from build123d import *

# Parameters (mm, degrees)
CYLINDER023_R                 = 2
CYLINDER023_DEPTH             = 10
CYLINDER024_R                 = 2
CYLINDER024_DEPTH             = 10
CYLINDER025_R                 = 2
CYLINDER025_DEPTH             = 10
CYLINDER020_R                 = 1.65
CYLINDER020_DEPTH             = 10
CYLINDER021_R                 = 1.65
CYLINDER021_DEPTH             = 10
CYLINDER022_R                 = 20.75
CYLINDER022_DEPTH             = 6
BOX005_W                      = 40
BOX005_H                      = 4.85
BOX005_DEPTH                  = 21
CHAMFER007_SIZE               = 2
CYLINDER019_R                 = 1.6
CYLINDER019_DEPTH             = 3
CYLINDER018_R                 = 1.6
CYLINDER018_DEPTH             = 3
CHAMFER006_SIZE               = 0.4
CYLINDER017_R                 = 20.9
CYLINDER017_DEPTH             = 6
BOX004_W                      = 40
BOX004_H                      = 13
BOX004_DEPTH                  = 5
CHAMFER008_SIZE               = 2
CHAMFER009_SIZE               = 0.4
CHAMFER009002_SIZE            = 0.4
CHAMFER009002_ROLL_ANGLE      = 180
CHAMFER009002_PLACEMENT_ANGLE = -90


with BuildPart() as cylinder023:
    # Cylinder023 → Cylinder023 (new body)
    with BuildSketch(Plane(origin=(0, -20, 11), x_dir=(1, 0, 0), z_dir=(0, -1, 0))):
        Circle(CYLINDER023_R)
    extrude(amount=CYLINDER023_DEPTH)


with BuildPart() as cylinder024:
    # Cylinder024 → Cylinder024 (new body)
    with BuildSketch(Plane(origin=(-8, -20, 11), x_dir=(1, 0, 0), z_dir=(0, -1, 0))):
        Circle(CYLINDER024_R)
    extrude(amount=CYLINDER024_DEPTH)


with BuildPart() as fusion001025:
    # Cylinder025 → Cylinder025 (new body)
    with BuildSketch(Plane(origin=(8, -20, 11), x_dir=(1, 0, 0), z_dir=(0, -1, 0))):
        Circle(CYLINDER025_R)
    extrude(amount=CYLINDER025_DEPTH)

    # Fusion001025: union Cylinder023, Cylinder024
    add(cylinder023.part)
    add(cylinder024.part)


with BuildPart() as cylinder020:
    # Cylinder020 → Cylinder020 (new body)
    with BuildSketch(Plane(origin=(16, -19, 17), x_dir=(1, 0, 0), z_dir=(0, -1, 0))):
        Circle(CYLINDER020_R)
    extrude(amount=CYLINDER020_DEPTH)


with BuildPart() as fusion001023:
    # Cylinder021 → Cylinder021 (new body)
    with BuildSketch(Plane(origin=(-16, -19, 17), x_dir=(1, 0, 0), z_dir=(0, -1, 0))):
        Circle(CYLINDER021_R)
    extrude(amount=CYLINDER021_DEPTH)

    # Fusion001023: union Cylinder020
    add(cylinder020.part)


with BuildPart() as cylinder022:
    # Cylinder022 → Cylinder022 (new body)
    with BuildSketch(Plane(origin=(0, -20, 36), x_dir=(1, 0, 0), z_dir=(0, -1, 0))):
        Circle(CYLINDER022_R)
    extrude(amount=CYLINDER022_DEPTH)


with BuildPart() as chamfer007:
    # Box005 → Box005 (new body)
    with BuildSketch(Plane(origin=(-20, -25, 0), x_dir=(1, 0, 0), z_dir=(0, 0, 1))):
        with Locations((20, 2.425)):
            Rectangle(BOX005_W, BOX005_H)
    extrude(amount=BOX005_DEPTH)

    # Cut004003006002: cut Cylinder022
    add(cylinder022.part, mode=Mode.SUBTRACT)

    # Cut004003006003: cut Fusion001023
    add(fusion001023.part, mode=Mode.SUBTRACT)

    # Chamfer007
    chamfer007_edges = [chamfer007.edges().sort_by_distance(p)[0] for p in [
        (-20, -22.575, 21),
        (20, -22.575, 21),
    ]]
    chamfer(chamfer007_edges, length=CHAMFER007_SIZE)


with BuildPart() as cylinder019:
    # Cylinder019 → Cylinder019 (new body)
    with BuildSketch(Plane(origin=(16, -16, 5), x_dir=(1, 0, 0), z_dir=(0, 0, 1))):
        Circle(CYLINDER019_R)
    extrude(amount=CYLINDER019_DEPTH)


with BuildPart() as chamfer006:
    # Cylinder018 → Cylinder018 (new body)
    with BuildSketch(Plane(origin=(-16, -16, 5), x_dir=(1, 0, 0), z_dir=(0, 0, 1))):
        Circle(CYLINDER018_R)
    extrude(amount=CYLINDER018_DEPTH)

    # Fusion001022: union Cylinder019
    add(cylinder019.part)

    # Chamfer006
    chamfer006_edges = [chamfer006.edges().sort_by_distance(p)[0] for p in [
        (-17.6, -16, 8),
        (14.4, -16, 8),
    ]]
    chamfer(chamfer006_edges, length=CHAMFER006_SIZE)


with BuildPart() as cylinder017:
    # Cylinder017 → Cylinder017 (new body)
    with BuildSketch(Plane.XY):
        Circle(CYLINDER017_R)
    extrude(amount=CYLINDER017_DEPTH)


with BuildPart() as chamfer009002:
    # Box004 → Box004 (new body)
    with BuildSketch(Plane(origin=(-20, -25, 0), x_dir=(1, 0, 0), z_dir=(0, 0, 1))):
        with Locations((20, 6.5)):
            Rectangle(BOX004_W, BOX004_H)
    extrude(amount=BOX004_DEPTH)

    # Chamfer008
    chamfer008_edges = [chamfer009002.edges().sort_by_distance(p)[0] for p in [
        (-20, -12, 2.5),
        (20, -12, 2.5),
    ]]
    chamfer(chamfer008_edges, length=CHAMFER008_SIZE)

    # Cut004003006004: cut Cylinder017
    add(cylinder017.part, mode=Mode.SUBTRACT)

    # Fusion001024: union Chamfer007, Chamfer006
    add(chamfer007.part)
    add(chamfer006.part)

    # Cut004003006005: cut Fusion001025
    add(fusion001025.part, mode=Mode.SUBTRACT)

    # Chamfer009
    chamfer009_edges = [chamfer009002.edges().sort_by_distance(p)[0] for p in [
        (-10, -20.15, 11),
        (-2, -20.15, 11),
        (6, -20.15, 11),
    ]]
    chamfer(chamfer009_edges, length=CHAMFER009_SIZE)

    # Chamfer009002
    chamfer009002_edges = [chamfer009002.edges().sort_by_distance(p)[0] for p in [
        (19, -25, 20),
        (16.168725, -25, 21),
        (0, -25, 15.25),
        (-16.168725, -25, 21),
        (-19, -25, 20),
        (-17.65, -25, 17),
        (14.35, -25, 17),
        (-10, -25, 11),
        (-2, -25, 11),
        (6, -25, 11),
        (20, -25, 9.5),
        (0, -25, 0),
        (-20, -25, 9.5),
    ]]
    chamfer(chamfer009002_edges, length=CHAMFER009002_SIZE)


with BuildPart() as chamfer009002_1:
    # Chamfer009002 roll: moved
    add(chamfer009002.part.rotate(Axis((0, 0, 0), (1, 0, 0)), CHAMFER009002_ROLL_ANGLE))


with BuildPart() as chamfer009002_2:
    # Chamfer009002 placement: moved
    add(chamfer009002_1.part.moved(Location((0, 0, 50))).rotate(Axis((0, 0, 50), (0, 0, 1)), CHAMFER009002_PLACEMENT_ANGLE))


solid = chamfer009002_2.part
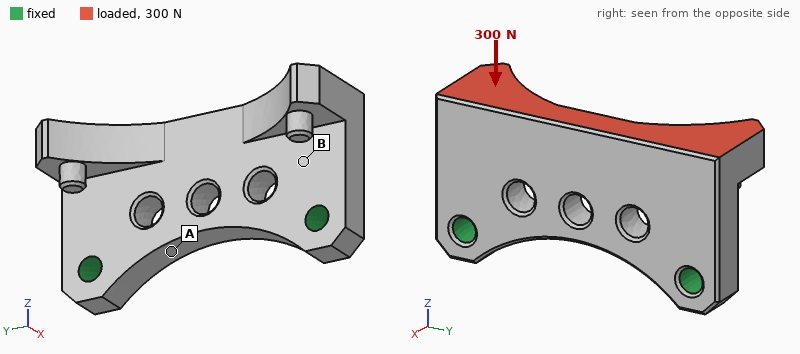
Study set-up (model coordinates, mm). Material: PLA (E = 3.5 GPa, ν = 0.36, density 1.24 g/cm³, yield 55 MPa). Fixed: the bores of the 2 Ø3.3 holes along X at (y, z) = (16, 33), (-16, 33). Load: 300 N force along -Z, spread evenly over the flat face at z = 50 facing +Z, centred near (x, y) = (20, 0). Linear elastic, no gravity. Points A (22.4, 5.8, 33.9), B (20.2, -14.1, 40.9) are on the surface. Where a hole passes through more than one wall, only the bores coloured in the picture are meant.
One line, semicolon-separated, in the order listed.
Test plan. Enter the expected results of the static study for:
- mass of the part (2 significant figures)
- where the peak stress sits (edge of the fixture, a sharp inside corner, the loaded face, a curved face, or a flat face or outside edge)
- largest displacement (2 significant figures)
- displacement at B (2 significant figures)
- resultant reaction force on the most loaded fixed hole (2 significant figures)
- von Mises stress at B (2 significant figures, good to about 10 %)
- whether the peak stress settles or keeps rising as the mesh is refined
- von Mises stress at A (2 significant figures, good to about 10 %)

4.8 g; edge of the fixture; 0.19 mm; 0.038 mm; 160 N; 8.9 MPa; keeps rising; 2.9 MPa
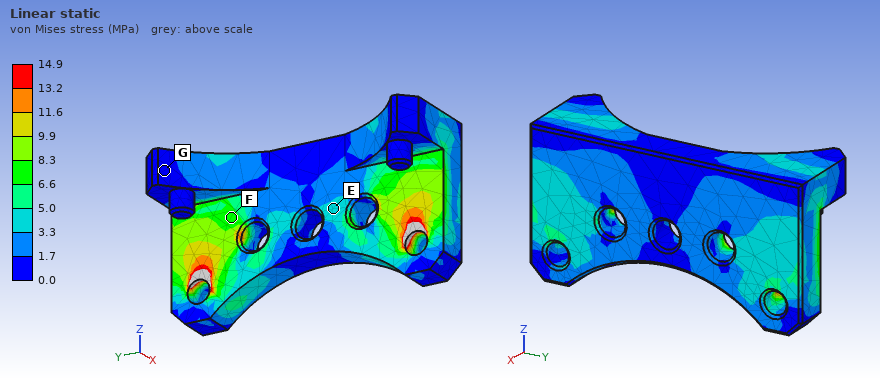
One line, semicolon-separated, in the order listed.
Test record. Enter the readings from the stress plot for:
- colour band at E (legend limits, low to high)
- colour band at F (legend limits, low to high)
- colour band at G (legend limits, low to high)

3.3 to 5.0 MPa; 6.6 to 8.3 MPa; 0.0 to 1.7 MPa
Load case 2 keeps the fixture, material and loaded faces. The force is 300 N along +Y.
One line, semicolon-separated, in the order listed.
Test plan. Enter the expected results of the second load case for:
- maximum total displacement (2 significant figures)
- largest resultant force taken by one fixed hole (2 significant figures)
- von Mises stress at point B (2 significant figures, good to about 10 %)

95 µm; 210 N; 5.2 MPa
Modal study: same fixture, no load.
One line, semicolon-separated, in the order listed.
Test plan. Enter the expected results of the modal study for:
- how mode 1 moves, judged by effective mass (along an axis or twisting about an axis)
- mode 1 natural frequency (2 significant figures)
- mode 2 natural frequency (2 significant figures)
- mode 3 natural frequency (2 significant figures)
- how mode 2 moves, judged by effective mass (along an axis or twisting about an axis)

along X; 2500 Hz; 4000 Hz; 5700 Hz; twisting about Z
